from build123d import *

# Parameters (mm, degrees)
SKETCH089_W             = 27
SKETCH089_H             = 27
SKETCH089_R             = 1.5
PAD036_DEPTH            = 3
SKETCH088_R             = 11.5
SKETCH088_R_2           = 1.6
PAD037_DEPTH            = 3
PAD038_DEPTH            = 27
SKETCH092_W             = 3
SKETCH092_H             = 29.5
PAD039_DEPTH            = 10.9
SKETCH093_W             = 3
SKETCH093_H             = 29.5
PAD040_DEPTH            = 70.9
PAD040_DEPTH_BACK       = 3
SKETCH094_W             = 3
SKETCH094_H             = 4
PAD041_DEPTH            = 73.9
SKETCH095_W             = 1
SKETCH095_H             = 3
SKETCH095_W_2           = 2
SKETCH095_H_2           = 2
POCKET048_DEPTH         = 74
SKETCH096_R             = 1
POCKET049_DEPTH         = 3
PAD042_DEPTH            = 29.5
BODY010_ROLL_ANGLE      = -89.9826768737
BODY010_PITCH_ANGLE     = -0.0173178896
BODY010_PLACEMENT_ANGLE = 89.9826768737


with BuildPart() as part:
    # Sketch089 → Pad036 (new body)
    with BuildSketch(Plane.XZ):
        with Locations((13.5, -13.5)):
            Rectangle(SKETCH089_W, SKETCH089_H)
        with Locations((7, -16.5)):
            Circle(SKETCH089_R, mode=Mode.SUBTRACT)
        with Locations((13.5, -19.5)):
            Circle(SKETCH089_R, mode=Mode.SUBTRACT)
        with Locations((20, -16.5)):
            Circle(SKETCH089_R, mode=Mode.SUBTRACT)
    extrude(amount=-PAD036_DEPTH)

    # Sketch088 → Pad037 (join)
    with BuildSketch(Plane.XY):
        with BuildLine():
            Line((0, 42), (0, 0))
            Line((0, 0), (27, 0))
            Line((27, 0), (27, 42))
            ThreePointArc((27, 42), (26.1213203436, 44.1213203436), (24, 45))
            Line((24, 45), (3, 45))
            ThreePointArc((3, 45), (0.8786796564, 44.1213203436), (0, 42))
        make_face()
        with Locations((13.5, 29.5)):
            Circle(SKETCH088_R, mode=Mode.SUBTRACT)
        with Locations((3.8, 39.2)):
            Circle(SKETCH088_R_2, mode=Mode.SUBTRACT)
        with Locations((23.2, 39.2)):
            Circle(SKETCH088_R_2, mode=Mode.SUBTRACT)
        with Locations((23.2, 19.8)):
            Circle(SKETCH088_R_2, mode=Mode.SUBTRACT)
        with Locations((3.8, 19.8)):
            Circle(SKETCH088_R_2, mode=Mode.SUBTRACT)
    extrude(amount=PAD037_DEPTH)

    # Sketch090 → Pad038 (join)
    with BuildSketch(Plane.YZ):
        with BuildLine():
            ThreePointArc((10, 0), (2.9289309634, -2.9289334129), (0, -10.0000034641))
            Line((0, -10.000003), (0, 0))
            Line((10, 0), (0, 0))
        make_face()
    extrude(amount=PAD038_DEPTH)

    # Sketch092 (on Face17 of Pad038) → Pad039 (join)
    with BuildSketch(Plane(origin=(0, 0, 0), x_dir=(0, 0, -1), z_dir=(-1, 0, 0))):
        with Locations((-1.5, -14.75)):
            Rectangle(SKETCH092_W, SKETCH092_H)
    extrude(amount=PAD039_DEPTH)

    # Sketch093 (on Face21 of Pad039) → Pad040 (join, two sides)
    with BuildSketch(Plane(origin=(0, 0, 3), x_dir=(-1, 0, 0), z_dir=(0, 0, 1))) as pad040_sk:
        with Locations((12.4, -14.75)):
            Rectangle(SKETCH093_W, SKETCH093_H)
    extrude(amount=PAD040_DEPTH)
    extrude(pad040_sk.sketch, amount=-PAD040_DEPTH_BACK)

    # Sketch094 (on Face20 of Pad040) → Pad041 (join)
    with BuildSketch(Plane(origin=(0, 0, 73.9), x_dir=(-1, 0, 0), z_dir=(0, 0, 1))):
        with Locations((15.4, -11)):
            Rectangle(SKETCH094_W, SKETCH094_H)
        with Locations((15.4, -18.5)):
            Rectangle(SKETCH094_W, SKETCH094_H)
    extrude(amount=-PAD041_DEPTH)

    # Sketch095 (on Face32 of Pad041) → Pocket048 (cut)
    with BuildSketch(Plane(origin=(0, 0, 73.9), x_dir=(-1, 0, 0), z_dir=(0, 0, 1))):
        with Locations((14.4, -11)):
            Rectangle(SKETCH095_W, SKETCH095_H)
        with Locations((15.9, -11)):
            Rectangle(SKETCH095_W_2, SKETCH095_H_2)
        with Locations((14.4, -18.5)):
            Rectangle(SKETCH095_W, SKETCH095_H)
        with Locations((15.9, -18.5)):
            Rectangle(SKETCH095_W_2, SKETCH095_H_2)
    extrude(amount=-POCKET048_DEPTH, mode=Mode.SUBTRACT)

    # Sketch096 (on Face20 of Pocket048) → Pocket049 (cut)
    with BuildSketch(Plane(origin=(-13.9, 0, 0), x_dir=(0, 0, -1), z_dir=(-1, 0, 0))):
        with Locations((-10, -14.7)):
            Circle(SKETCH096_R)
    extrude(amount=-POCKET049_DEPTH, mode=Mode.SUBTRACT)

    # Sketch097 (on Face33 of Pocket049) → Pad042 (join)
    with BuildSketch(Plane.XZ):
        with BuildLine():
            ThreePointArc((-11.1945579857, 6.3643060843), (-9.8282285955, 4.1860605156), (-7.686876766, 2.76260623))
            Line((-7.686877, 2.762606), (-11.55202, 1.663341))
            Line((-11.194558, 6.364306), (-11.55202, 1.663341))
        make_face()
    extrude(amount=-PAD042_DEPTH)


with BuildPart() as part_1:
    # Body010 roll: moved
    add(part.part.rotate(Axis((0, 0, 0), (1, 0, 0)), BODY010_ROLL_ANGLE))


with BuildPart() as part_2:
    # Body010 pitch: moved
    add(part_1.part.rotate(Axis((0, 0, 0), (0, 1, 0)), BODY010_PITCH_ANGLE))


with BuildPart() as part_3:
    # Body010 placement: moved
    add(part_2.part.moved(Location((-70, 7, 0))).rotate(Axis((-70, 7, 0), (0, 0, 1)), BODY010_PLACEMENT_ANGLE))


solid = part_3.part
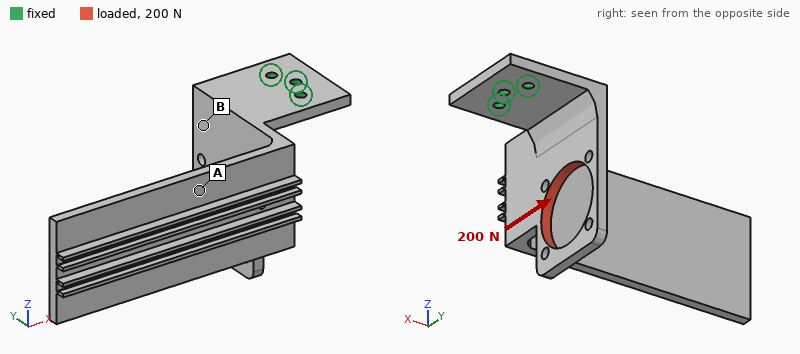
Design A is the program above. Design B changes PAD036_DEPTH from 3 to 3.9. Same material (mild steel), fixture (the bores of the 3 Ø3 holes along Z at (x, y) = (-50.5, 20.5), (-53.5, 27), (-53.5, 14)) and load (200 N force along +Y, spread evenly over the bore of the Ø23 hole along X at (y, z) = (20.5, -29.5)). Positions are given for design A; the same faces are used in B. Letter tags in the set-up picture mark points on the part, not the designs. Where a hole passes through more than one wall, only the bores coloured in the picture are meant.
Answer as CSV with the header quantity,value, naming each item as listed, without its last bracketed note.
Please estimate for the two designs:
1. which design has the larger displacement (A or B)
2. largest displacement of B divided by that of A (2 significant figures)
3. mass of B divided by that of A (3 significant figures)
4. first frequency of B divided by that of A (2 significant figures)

quantity,value
which design has the larger displacement,A
largest displacement of B divided by that of A,0.65
mass of B divided by that of A,1.04
first frequency of B divided by that of A,1.2
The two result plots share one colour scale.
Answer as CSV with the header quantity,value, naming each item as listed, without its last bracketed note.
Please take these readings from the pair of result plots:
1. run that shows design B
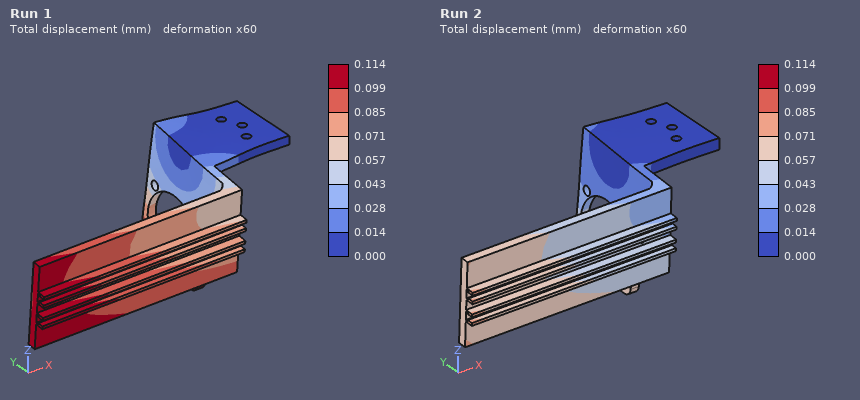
quantity,value
run that shows design B,Run 2
